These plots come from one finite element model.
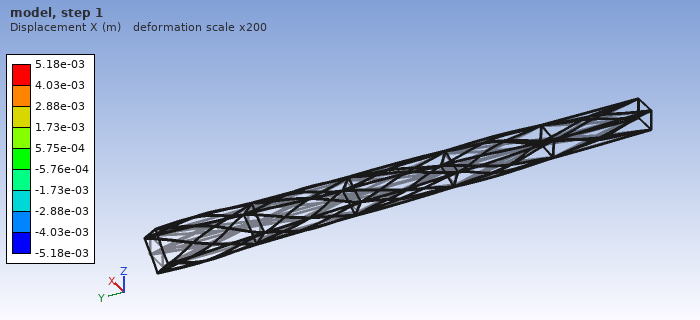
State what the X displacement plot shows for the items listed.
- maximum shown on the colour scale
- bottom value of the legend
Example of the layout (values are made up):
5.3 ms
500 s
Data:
5.18e-03 m
-5.18e-03 m
